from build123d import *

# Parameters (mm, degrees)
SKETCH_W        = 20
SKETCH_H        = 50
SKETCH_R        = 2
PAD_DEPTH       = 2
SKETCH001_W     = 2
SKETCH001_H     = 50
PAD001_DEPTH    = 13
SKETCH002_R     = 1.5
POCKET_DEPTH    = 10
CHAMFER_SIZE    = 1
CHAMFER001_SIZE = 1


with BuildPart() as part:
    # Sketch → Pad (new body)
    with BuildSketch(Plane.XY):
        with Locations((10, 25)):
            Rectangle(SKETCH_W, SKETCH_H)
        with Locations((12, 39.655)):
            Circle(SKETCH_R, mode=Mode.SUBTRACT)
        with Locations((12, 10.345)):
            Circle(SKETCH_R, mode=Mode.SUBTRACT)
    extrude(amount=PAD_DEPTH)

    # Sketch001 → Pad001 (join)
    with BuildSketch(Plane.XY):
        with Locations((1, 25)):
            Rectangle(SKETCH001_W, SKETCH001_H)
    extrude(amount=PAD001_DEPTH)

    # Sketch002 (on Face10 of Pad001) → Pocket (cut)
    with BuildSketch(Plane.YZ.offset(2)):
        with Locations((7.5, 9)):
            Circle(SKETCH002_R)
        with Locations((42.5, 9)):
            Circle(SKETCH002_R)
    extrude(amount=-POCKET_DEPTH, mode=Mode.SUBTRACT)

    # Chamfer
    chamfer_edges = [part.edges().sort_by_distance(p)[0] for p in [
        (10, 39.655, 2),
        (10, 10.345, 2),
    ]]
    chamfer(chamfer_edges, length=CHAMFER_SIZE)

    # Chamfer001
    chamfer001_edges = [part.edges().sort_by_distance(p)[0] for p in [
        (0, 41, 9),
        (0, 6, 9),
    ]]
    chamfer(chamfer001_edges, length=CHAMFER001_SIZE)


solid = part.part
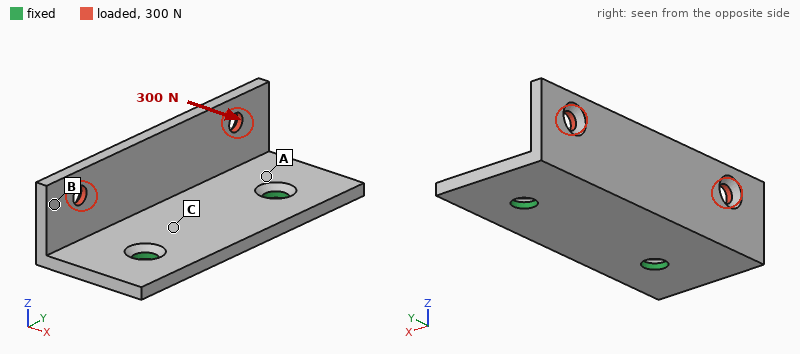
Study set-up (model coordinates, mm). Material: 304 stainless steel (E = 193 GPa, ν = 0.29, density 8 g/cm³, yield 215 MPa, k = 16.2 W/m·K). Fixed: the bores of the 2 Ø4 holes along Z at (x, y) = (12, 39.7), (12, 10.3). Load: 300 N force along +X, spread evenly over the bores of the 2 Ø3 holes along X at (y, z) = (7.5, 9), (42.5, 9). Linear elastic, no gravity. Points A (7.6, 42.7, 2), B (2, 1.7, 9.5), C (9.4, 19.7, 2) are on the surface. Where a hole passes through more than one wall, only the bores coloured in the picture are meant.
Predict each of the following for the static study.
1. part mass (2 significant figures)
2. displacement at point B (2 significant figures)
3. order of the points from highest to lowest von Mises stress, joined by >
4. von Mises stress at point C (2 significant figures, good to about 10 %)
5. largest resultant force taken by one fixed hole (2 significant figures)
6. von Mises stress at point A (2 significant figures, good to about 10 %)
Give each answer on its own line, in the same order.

24 g
60 µm
A > C > B
47 MPa
150 N
91 MPa
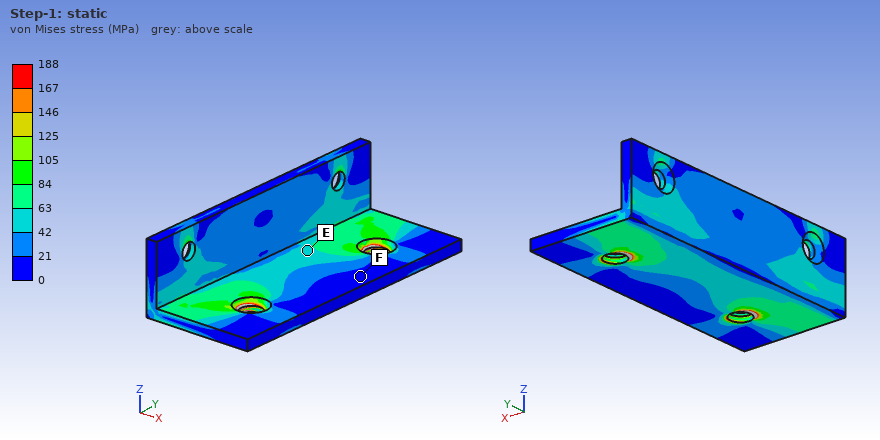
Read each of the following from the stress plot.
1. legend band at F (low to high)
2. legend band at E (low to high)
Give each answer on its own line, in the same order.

0 to 21 MPa
42 to 63 MPa
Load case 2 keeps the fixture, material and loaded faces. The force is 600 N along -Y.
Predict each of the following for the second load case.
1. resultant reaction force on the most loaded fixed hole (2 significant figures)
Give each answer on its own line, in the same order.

390 N
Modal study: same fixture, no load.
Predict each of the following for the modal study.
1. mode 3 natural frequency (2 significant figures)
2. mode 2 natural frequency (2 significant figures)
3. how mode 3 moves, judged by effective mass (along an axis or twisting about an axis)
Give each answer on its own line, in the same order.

9600 Hz
5000 Hz
along Z
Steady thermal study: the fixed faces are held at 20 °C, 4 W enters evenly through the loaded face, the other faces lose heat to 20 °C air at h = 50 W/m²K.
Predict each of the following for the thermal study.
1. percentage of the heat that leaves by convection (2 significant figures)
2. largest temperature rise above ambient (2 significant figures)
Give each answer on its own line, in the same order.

59 %
53 K
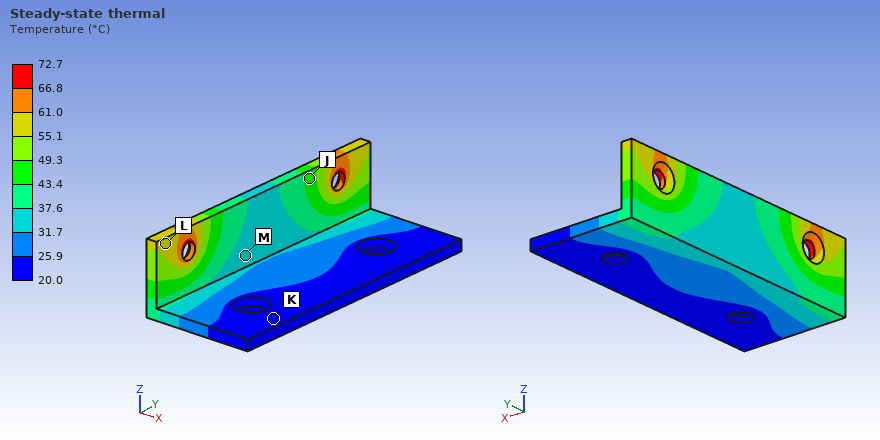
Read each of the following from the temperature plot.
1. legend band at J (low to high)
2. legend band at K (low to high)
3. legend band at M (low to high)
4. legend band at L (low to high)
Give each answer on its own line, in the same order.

43.4 to 49.3 °C
20.0 to 25.9 °C
31.7 to 37.6 °C
55.1 to 61.0 °C
